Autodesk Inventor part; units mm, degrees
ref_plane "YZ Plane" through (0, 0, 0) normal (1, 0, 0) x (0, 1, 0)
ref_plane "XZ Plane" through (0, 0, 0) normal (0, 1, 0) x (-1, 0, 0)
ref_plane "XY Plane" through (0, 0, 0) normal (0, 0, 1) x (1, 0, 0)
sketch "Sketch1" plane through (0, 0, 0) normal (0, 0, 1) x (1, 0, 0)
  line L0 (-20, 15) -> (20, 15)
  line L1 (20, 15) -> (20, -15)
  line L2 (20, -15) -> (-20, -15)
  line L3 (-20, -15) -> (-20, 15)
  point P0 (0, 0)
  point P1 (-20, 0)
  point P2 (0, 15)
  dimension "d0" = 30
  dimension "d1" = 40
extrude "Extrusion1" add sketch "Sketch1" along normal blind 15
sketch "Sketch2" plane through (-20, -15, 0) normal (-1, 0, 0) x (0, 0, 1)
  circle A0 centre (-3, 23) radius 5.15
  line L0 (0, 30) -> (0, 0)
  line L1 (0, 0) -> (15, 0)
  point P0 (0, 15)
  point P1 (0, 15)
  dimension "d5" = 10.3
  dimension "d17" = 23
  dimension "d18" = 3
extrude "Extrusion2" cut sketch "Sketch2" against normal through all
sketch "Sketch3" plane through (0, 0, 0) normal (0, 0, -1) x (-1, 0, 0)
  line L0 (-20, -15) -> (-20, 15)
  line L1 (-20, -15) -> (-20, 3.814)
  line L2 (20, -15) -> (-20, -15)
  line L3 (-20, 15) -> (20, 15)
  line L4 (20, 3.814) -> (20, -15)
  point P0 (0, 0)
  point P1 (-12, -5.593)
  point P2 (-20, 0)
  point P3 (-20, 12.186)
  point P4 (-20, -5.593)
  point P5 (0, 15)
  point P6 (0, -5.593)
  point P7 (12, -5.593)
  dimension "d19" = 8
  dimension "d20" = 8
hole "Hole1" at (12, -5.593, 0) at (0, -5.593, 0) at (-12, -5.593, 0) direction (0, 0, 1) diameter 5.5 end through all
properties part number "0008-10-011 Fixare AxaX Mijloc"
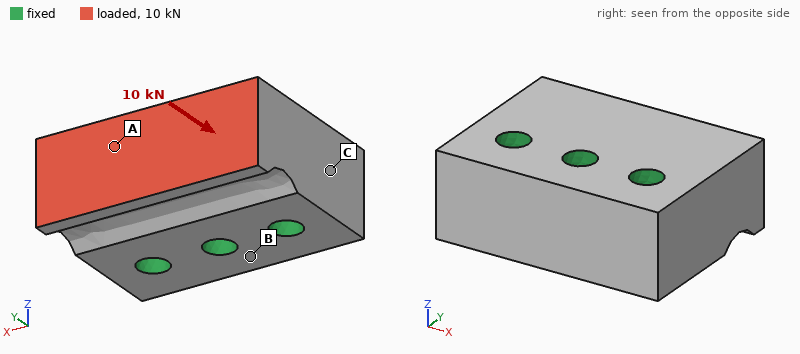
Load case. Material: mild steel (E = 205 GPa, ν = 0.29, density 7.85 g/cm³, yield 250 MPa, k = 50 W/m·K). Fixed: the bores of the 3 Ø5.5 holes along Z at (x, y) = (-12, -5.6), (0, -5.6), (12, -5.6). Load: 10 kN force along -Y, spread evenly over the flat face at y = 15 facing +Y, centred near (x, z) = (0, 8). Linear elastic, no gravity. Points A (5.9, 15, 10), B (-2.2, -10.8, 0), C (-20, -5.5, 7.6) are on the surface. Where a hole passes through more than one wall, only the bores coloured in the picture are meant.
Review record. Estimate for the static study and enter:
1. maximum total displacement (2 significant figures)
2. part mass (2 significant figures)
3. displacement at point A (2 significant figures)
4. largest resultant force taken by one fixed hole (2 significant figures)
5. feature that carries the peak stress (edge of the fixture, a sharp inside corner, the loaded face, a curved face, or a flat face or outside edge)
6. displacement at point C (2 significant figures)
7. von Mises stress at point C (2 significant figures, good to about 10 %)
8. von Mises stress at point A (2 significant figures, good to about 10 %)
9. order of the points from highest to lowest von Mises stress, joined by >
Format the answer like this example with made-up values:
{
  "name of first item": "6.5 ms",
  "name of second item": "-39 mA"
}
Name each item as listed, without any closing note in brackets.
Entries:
{
  "maximum total displacement": "2.8 µm",
  "part mass": "130 g",
  "displacement at point A": "1.6 µm",
  "largest resultant force taken by one fixed hole": "3.7 kN",
  "feature that carries the peak stress": "a curved face",
  "displacement at point C": "0.49 µm",
  "von Mises stress at point C": "8.7 MPa",
  "von Mises stress at point A": "20 MPa",
  "order of the points from highest to lowest von Mises stress, joined by >": "A > C > B"
}
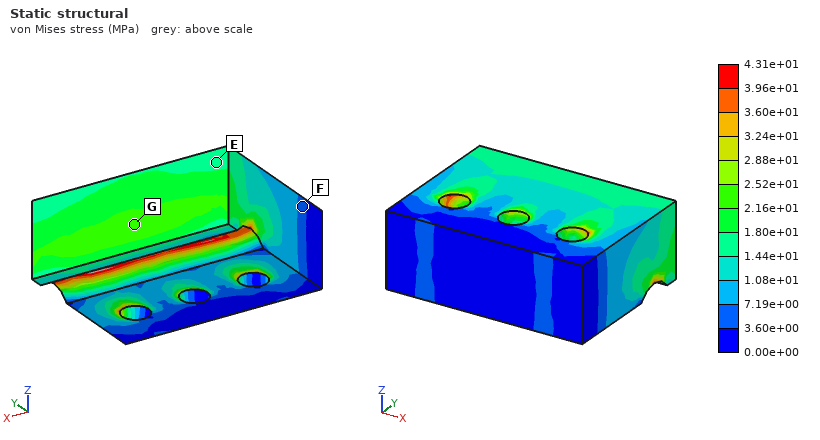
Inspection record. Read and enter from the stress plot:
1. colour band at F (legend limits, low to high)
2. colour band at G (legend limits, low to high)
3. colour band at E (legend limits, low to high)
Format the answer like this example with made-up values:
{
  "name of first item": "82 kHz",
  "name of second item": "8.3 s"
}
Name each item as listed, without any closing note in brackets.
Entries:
{
  "colour band at F": "3.60e+00 to 7.19e+00 MPa",
  "colour band at G": "2.16e+01 to 2.52e+01 MPa",
  "colour band at E": "1.44e+01 to 1.80e+01 MPa"
}
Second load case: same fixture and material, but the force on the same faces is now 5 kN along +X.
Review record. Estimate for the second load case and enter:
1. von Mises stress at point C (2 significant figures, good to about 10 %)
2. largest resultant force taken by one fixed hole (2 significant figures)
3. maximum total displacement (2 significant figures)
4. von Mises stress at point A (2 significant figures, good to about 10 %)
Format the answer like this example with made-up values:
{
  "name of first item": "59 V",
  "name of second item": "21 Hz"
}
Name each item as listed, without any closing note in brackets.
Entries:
{
  "von Mises stress at point C": "16 MPa",
  "largest resultant force taken by one fixed hole": "3.8 kN",
  "maximum total displacement": "5.1 µm",
  "von Mises stress at point A": "16 MPa"
}
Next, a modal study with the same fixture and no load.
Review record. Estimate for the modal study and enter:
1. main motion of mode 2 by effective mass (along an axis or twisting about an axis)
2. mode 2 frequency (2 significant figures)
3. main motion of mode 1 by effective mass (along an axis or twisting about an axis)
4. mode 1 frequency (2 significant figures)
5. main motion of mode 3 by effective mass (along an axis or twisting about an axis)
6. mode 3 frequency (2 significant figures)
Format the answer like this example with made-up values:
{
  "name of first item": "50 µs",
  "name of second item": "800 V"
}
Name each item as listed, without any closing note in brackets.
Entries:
{
  "main motion of mode 2 by effective mass": "twisting about Y",
  "mode 2 frequency": "30 kHz",
  "main motion of mode 1 by effective mass": "along Z",
  "mode 1 frequency": "24 kHz",
  "main motion of mode 3 by effective mass": "along X",
  "mode 3 frequency": "32 kHz"
}
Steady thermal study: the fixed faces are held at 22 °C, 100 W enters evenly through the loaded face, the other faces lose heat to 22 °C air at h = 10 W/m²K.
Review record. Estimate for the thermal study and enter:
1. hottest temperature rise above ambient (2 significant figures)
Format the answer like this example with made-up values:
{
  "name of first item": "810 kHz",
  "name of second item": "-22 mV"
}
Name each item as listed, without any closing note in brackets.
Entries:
{
  "hottest temperature rise above ambient": "72 K"
}
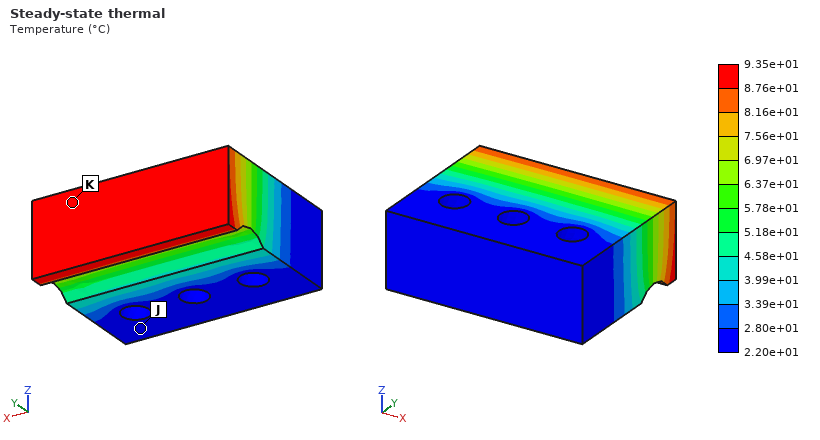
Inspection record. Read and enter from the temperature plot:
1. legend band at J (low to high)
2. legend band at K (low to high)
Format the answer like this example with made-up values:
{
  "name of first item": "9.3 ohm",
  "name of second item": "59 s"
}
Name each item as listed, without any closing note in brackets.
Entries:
{
  "legend band at J": "2.20e+01 to 2.80e+01 °C",
  "legend band at K": "8.76e+01 to 9.35e+01 °C"
}
